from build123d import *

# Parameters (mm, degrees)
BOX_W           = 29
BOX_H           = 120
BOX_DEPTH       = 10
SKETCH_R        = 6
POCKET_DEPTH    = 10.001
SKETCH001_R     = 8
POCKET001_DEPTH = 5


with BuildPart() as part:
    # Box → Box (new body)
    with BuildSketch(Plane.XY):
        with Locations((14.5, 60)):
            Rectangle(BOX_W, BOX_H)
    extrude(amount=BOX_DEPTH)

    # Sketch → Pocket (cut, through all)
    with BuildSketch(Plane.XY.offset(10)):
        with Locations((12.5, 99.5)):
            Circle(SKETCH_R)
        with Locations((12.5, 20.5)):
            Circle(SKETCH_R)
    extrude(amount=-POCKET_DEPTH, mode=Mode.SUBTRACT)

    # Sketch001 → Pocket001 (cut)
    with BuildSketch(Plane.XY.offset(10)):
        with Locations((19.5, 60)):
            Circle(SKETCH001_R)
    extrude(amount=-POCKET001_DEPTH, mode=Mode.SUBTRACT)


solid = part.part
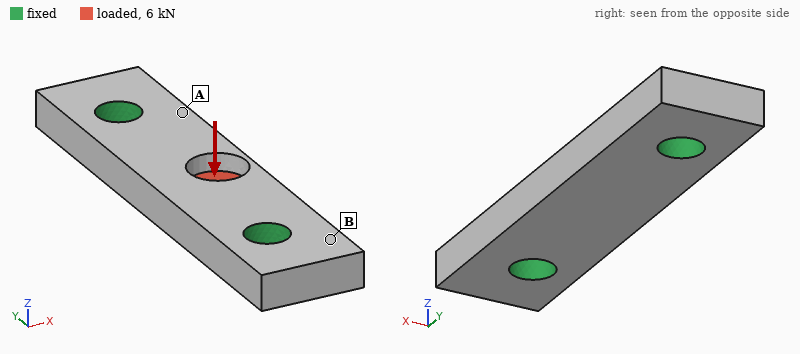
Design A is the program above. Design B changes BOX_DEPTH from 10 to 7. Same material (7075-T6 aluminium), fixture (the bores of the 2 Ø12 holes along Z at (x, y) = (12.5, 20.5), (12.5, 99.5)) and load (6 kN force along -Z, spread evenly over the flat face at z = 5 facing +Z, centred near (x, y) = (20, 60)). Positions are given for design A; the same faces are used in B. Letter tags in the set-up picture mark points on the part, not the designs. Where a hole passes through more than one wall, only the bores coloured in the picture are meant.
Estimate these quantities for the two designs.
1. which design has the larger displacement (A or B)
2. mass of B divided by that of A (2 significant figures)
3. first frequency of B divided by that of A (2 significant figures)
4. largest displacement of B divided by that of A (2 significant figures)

B
0.71
0.74
2.4
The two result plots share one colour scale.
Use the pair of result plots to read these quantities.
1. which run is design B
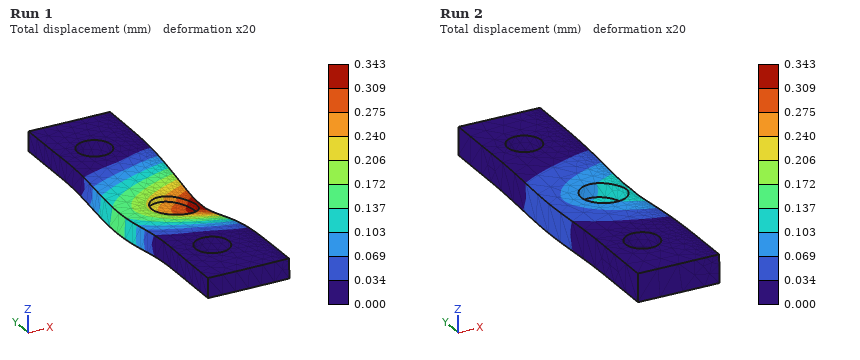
Run 1
